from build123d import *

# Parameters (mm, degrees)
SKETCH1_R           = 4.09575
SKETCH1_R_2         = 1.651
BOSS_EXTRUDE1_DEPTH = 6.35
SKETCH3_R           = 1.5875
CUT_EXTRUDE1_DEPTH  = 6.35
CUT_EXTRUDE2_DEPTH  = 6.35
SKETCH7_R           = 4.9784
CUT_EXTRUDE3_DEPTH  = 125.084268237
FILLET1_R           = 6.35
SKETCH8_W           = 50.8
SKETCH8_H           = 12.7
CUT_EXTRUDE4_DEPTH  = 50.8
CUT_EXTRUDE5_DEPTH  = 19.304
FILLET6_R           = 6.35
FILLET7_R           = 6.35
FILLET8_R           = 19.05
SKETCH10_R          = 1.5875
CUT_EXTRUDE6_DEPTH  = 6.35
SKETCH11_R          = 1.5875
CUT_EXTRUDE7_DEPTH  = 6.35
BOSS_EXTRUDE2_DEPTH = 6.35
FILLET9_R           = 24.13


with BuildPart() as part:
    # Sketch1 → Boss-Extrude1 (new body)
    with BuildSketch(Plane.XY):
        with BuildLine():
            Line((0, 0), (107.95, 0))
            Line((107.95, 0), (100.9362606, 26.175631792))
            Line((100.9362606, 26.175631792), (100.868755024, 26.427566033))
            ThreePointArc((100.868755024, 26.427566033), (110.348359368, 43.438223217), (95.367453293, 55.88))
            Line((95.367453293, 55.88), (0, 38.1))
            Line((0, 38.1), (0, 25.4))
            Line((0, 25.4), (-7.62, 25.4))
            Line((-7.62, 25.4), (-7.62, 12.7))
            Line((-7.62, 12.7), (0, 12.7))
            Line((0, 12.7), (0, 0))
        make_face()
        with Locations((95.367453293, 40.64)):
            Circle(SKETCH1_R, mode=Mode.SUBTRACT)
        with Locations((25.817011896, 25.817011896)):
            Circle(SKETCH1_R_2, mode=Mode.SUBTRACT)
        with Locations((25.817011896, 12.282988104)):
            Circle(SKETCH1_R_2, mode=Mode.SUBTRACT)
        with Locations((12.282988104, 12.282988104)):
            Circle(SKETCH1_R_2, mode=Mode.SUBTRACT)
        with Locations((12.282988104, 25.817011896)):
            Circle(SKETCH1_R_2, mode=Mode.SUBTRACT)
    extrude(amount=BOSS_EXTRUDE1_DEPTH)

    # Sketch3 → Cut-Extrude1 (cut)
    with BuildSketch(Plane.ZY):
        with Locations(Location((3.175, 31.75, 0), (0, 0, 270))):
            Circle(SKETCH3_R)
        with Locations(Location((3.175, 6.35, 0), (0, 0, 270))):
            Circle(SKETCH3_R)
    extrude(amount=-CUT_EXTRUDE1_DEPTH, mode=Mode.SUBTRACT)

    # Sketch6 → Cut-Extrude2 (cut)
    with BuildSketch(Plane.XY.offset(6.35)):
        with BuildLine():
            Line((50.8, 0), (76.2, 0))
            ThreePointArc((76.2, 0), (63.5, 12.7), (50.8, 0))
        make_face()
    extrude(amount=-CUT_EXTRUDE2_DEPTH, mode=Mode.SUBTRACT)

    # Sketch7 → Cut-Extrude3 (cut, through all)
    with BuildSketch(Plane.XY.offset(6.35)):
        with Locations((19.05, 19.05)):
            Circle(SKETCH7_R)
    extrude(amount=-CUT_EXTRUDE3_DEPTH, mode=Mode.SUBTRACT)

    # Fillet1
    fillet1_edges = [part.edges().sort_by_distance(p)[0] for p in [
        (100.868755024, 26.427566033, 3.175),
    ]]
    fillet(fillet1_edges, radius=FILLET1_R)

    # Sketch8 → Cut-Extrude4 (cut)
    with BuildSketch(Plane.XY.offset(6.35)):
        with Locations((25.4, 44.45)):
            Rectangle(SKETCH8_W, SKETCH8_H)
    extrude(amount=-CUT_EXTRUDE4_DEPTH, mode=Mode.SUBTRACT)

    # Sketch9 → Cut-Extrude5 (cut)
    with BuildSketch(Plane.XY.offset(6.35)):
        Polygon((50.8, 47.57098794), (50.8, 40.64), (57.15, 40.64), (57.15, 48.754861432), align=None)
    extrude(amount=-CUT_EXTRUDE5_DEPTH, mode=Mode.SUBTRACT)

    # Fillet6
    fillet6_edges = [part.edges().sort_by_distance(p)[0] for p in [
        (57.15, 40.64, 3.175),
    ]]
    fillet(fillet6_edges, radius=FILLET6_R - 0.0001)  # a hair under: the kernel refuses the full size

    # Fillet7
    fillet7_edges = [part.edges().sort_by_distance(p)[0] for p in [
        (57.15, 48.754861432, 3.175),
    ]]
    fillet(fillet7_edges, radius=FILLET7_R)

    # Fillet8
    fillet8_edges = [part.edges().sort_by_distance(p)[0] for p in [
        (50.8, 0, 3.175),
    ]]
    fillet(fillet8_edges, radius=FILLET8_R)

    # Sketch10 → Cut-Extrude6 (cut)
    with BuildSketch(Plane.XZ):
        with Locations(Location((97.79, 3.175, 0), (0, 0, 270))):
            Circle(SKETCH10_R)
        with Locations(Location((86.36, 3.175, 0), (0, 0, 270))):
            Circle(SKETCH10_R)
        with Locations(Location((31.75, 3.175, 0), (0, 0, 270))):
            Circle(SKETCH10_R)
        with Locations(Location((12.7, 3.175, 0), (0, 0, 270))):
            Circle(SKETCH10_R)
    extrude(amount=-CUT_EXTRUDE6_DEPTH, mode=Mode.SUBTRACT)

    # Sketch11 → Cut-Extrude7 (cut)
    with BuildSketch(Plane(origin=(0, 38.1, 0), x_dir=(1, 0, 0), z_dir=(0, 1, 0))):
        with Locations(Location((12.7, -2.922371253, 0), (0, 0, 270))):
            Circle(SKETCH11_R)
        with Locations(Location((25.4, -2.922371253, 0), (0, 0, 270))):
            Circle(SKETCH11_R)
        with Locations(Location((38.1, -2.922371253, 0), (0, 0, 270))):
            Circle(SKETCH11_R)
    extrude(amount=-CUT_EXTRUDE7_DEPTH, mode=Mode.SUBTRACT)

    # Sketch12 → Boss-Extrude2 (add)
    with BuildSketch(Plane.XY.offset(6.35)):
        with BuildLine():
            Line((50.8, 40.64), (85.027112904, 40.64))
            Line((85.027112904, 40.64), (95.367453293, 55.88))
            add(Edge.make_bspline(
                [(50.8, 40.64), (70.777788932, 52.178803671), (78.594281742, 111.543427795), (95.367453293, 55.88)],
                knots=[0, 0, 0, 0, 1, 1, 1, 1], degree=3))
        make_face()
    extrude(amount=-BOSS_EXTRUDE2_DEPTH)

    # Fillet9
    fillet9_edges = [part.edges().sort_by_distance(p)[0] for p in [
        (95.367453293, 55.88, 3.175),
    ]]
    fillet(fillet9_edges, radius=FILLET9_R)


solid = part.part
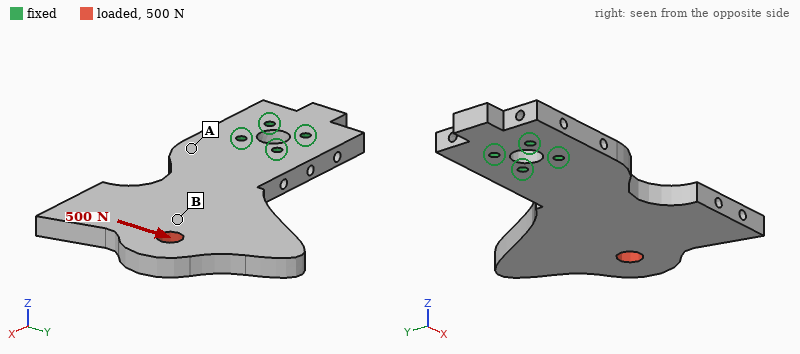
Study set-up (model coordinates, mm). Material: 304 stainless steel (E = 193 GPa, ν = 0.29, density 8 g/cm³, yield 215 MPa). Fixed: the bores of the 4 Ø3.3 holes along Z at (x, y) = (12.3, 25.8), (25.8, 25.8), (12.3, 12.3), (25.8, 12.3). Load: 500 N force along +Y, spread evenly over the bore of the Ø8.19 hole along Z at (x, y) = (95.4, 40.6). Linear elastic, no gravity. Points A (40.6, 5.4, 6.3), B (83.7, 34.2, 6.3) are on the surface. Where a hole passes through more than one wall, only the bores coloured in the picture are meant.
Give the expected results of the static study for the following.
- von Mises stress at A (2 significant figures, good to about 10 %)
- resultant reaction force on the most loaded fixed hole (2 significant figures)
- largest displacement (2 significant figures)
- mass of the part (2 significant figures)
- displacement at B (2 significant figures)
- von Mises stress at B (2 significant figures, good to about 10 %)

14 MPa
1.4 kN
29 µm
250 g
18 µm
5.0 MPa
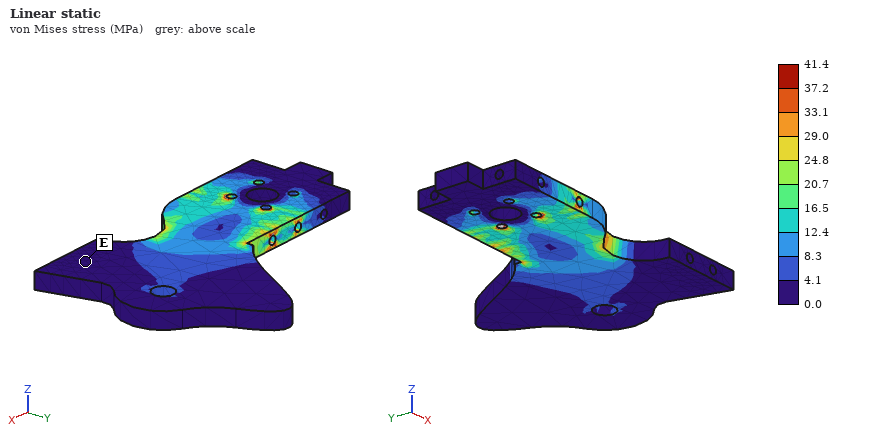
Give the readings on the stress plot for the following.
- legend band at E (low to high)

0.0 to 4.1 MPa
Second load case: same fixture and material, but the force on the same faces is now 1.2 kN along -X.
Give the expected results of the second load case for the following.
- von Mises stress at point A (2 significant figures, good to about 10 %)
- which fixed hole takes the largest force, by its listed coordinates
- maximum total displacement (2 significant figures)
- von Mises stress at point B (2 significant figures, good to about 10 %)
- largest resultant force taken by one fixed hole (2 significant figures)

8.0 MPa
(25.8, 25.8)
24 µm
7.7 MPa
1.5 kN
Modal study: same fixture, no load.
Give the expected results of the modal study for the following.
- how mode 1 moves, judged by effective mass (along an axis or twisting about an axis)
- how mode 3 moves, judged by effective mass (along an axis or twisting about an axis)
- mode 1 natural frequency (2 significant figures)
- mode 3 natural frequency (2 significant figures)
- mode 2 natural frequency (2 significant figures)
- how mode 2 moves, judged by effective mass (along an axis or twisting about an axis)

along Z
along Y
560 Hz
2200 Hz
1400 Hz
twisting about X
